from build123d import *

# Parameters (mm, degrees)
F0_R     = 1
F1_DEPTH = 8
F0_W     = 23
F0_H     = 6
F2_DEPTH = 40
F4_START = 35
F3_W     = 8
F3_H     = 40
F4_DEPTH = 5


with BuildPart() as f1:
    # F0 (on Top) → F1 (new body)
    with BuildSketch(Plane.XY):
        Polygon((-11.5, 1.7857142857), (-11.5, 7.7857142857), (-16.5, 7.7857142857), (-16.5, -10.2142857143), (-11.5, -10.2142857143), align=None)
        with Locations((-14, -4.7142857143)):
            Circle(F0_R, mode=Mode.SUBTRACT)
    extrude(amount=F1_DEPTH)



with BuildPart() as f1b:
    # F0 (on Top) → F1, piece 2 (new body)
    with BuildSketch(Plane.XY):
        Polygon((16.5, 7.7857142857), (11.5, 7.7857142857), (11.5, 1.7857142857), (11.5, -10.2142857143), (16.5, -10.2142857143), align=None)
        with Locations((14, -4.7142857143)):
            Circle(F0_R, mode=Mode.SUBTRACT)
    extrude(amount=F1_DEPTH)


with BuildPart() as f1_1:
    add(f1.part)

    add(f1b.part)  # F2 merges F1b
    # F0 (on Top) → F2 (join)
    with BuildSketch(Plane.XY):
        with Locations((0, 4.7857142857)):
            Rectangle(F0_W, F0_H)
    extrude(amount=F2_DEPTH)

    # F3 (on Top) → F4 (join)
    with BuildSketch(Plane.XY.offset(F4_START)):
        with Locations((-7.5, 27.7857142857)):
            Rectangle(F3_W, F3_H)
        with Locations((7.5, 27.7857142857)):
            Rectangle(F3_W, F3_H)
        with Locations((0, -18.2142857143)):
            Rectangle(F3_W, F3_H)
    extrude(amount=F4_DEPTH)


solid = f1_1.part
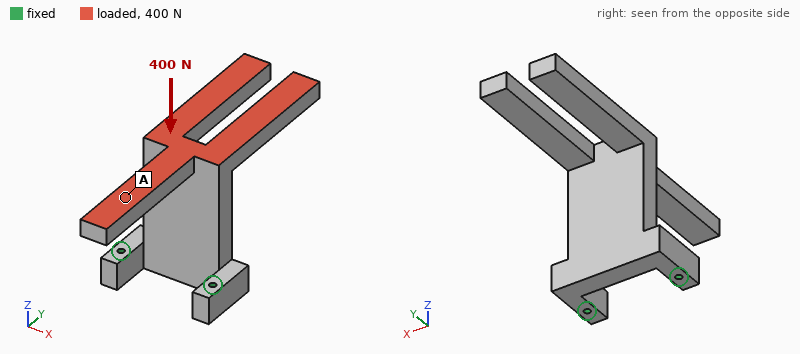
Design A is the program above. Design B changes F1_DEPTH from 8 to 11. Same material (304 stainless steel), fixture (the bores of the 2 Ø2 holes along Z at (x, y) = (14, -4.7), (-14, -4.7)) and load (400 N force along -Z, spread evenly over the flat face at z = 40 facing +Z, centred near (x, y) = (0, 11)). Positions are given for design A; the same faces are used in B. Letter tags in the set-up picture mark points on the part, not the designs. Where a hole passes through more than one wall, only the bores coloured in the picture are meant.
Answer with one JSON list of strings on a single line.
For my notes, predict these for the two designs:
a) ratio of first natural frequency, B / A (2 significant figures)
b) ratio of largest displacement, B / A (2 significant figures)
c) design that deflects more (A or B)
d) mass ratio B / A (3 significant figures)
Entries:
["1.2", "0.84", "A", "1.04"]
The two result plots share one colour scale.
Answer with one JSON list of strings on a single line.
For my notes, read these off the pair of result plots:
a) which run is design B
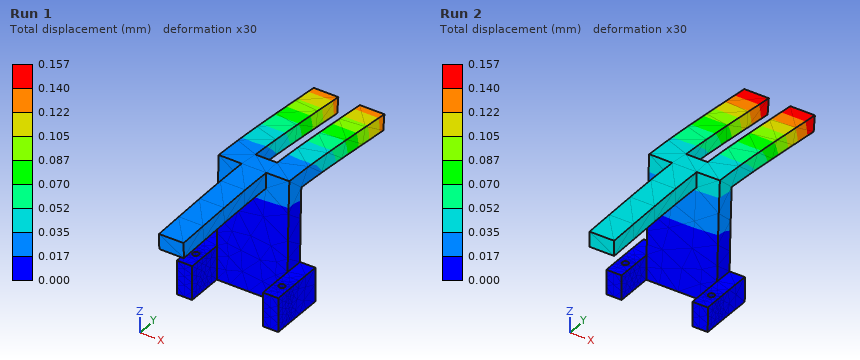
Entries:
["Run 1"]
